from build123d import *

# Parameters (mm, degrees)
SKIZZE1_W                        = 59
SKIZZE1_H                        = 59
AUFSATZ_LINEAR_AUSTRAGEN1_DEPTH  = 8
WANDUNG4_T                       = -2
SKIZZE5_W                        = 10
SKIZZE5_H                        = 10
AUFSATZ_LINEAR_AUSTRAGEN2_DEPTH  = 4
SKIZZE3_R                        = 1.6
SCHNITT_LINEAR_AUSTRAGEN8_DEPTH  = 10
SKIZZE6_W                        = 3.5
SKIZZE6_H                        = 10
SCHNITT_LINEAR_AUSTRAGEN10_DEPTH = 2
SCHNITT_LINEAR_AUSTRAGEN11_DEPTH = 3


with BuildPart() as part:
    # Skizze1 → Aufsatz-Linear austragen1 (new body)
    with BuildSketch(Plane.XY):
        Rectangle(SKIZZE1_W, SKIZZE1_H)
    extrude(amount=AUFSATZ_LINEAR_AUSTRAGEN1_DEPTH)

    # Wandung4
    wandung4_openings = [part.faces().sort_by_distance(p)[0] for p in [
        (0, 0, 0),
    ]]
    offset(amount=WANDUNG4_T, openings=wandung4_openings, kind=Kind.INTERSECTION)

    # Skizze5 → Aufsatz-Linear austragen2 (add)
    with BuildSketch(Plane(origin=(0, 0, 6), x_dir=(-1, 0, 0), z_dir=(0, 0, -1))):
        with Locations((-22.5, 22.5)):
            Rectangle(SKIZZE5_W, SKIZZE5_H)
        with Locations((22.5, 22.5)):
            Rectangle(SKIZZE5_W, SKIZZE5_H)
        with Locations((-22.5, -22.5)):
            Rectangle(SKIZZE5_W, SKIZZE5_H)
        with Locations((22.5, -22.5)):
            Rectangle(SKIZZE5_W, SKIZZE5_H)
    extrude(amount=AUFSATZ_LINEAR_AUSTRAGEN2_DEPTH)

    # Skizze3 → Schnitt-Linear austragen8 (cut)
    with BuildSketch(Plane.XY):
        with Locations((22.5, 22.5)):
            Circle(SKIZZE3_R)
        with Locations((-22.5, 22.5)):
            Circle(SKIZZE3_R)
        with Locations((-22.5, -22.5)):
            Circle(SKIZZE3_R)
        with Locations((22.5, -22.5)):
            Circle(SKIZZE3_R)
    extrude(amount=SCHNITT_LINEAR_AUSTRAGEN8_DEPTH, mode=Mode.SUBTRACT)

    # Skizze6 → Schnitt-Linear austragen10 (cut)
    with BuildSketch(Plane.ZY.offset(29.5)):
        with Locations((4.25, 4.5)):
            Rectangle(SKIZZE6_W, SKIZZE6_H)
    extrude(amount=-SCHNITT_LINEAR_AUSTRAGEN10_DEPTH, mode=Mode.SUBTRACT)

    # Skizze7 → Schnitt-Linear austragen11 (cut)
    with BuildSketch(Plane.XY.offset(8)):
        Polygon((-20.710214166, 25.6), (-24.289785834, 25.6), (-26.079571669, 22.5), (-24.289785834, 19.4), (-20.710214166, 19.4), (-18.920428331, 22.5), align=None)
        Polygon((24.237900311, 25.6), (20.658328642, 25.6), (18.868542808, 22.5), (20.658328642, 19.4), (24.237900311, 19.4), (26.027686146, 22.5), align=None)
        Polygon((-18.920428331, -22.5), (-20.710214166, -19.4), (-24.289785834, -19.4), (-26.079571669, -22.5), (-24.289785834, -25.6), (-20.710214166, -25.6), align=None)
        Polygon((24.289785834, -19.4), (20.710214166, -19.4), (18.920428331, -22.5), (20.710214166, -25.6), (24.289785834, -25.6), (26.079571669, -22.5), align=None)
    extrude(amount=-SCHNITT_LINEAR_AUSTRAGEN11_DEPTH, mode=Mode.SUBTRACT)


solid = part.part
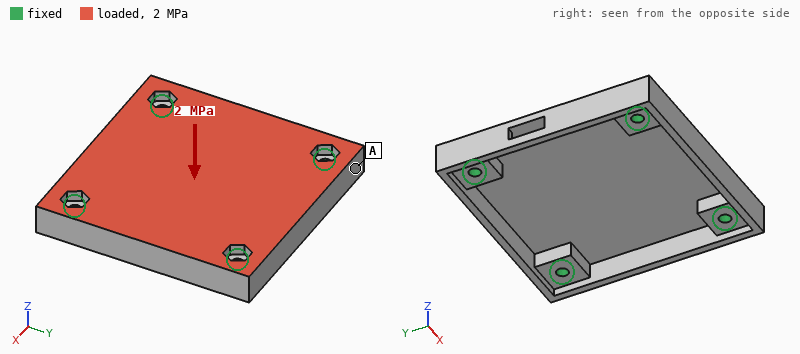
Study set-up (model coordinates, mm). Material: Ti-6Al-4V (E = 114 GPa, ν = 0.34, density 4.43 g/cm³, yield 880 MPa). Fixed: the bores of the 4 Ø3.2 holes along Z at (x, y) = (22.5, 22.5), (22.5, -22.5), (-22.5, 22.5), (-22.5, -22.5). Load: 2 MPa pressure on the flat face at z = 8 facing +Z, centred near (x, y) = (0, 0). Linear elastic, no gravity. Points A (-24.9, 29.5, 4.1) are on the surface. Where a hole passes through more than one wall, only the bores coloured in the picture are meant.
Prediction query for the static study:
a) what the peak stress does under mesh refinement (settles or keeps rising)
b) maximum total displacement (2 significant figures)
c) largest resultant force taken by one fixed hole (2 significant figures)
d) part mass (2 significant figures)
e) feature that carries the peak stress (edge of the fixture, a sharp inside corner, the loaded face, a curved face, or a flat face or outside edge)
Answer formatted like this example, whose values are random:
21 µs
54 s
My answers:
keeps rising
0.34 mm
2.4 kN
48 g
edge of the fixture
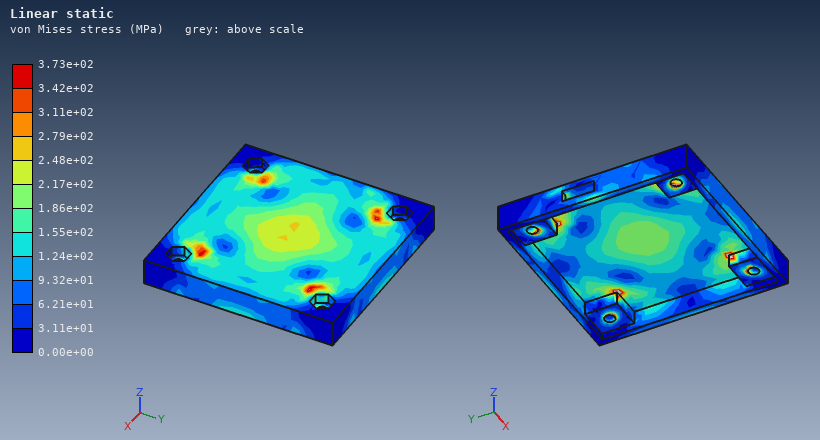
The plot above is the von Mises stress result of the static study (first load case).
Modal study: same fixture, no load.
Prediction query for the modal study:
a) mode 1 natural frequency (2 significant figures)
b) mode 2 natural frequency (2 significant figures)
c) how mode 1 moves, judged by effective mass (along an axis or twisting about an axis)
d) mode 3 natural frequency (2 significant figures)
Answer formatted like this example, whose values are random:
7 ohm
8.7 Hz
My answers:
5200 Hz
9700 Hz
along Z
9700 Hz
